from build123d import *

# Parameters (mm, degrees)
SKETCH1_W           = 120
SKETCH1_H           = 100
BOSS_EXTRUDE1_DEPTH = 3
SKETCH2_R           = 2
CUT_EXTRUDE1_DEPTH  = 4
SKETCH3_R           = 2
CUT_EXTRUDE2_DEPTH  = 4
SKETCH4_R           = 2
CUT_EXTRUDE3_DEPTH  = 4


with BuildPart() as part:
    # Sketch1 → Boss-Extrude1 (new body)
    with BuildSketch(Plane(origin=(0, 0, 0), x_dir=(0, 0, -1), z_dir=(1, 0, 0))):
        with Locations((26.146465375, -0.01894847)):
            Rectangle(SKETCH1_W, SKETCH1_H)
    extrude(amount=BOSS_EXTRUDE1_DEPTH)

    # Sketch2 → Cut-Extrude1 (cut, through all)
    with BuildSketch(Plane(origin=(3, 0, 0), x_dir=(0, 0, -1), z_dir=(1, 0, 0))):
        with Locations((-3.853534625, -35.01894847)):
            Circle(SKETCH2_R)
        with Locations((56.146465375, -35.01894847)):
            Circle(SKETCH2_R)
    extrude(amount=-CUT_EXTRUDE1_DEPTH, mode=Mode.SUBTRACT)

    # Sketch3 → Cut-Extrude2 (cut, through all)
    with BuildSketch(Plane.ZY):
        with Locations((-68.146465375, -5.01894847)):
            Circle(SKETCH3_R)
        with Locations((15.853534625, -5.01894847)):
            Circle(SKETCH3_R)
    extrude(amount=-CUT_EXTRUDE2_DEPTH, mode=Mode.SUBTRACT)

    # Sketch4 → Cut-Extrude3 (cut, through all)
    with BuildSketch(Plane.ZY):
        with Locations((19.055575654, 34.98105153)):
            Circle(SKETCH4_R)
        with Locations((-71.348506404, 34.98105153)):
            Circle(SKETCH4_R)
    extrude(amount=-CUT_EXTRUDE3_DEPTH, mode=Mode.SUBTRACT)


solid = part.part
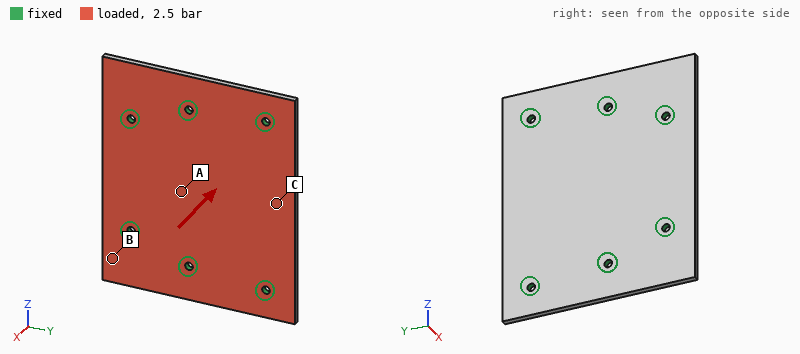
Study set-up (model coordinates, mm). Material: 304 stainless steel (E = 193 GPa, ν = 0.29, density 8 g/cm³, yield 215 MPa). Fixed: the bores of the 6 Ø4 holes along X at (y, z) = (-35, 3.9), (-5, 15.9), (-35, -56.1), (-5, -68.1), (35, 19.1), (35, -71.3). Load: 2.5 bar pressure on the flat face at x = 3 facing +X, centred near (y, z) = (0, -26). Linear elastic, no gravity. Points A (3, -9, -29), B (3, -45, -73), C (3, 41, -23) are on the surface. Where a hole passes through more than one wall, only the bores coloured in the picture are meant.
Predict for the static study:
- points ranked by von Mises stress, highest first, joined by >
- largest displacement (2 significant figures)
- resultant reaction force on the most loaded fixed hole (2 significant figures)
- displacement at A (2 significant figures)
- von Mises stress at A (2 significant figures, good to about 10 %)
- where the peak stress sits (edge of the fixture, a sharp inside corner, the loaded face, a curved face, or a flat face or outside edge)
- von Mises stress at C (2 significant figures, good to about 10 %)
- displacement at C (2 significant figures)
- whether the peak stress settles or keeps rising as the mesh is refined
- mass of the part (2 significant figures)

C > A > B
0.12 mm
520 N
0.056 mm
35 MPa
edge of the fixture
54 MPa
0.11 mm
keeps rising
290 g
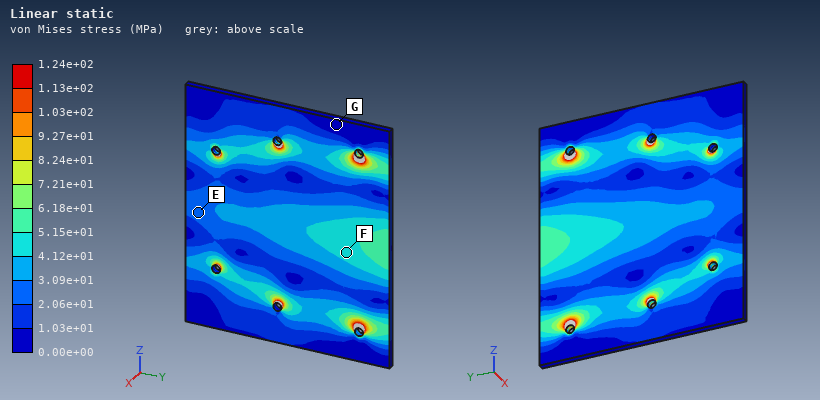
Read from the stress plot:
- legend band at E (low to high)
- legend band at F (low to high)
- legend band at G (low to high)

2.06e+01 to 3.09e+01 MPa
4.12e+01 to 5.15e+01 MPa
0.00e+00 to 1.03e+01 MPa
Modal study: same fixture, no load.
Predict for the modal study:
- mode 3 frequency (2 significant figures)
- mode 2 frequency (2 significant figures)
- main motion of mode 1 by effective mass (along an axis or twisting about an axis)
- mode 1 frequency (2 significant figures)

3300 Hz
3000 Hz
along X
1900 Hz
